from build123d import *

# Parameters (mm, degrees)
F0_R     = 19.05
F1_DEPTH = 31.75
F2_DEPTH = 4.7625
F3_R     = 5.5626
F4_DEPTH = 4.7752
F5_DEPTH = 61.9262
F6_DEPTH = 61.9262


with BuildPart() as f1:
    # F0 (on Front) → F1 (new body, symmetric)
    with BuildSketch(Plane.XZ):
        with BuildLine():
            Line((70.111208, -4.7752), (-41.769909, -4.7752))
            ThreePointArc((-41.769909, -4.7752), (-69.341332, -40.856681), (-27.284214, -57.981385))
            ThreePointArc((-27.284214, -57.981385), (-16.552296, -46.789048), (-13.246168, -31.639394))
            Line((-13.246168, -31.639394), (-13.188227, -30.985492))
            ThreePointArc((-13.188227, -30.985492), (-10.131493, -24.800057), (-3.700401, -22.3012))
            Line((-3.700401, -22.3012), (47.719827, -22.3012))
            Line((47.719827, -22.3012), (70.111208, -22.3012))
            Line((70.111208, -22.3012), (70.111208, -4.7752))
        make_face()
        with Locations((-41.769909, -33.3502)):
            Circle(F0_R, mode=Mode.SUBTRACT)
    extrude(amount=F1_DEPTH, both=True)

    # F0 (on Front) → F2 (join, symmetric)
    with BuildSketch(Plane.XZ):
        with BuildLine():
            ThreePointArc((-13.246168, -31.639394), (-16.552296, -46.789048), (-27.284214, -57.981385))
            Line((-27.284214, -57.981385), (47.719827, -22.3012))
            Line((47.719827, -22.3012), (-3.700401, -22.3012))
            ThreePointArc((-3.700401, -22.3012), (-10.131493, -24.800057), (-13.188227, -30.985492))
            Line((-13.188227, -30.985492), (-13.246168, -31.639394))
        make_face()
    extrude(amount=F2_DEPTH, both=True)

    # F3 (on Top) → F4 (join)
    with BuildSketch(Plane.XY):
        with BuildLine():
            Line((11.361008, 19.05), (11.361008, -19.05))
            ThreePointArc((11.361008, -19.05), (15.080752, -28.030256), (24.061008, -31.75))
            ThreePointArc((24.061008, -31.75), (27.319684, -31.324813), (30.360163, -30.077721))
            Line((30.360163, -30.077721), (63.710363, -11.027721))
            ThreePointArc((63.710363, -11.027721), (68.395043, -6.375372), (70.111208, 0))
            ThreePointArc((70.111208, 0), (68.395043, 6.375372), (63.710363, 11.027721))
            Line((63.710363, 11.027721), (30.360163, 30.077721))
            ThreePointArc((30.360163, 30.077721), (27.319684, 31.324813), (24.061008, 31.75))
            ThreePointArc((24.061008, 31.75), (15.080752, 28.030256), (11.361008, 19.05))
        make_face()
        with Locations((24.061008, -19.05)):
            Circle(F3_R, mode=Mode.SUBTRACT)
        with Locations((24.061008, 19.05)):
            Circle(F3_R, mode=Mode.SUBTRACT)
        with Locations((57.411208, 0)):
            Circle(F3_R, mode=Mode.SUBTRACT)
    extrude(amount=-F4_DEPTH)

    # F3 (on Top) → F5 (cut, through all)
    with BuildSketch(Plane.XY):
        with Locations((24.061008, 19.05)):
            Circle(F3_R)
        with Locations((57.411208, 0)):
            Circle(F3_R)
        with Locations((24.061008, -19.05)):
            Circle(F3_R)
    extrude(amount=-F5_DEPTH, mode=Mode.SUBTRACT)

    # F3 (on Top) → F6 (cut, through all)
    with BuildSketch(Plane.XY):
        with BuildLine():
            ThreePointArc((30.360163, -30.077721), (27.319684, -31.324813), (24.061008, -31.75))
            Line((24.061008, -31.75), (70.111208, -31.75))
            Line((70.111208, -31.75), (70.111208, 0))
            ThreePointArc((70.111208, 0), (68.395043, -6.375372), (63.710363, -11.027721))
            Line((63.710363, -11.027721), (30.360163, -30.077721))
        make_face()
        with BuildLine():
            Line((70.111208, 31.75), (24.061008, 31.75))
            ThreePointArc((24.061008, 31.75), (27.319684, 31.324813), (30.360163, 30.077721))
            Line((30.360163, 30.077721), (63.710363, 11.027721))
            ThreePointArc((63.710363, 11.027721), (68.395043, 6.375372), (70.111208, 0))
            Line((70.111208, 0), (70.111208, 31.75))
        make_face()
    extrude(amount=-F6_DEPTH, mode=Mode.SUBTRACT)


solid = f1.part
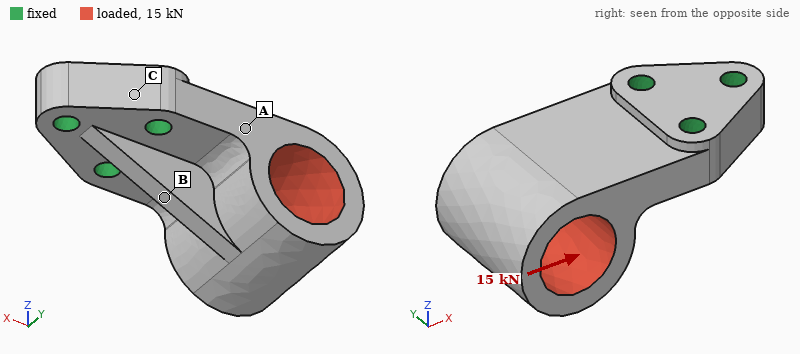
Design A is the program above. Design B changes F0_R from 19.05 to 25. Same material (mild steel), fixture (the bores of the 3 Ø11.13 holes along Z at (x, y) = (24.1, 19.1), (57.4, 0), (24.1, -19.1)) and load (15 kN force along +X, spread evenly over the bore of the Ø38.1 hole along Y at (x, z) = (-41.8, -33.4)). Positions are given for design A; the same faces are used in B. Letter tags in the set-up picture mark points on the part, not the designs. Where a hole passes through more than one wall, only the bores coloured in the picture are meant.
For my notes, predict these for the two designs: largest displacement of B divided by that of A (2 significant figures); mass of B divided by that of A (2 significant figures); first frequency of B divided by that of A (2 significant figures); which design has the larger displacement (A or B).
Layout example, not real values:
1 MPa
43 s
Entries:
2.8
0.73
0.92
B
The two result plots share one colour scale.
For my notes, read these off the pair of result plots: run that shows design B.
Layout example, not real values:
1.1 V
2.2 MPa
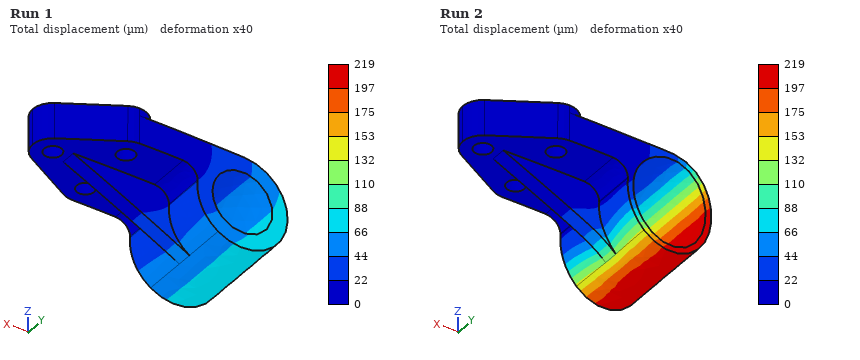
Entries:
Run 2
